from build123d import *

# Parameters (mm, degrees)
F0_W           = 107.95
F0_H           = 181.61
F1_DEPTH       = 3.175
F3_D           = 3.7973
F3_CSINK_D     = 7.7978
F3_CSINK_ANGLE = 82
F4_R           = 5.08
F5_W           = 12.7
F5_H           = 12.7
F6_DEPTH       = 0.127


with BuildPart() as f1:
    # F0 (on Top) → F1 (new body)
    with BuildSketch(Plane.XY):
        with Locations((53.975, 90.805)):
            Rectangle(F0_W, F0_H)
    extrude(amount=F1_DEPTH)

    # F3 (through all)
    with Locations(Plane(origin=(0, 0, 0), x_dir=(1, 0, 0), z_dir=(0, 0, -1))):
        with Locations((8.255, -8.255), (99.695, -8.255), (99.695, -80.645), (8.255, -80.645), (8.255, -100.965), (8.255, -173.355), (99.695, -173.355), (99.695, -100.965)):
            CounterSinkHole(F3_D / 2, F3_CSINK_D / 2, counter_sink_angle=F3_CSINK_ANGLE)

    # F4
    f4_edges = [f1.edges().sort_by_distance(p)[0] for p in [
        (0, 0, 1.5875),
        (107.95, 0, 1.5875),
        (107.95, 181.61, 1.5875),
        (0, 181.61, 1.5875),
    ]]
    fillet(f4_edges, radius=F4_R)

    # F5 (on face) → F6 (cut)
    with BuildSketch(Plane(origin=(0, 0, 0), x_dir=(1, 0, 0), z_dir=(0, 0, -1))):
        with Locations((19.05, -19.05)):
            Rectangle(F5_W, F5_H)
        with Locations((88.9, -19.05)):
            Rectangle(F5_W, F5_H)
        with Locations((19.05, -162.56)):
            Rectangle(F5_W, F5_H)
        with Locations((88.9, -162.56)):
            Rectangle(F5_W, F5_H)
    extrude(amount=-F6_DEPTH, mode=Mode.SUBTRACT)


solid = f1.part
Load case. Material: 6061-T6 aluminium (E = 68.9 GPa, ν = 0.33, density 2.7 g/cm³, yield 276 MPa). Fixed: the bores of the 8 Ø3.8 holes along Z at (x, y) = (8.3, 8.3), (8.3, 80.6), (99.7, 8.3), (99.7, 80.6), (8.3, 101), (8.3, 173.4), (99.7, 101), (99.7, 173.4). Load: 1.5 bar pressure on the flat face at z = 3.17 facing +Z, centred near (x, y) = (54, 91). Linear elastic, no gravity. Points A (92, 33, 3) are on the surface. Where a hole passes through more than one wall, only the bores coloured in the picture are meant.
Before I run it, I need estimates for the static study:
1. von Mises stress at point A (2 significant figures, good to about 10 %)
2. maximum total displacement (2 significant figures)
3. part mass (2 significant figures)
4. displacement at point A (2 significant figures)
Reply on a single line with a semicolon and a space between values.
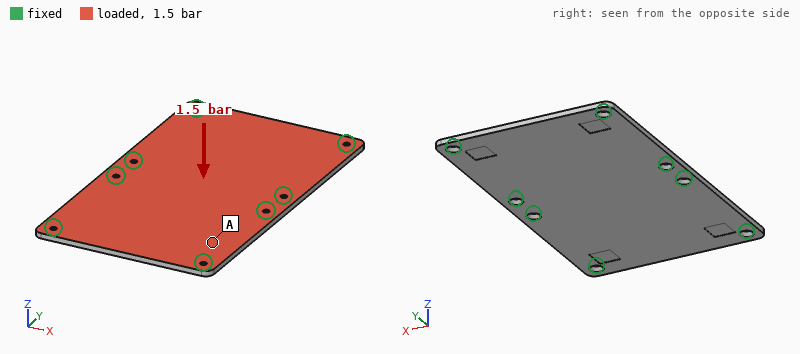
22 MPa; 0.36 mm; 170 g; 0.16 mm
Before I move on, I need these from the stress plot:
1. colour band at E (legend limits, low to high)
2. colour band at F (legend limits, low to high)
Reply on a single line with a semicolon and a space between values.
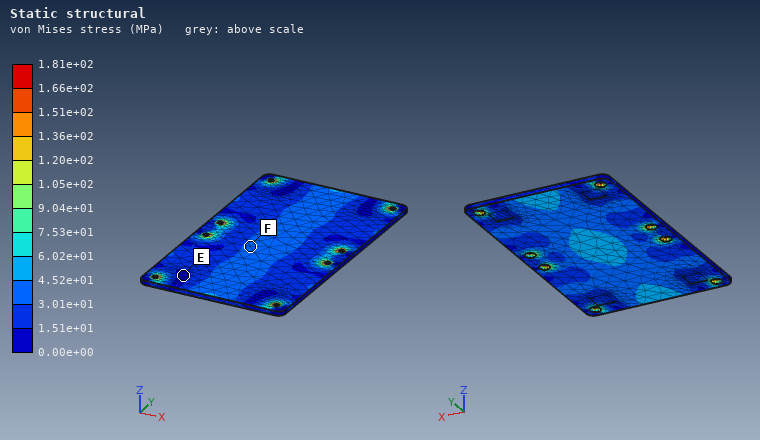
0.00e+00 to 1.51e+01 MPa; 3.01e+01 to 4.52e+01 MPa
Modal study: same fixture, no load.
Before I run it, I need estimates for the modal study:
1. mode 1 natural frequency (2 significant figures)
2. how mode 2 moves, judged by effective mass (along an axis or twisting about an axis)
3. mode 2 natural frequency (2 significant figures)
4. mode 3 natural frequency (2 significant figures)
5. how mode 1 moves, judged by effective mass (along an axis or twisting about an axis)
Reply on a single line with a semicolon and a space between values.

1300 Hz; twisting about X; 1400 Hz; 2100 Hz; along Z
